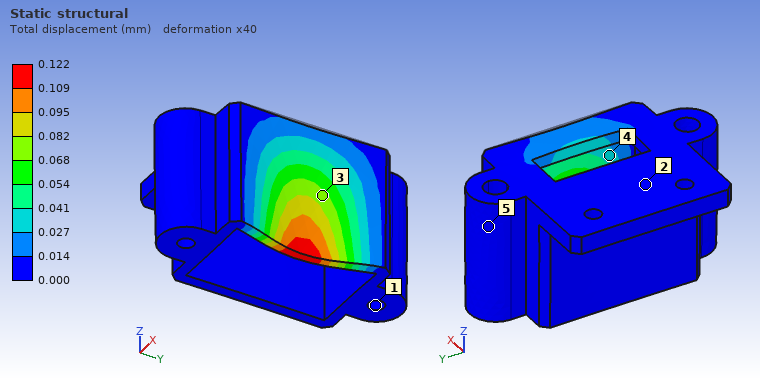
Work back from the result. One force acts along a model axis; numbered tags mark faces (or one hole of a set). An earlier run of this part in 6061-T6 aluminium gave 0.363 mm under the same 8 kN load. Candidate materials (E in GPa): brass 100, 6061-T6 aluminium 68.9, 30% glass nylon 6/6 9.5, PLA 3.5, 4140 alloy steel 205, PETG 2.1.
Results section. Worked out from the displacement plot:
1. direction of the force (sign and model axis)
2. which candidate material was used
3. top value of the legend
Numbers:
-X
4140 alloy steel
0.122 mm
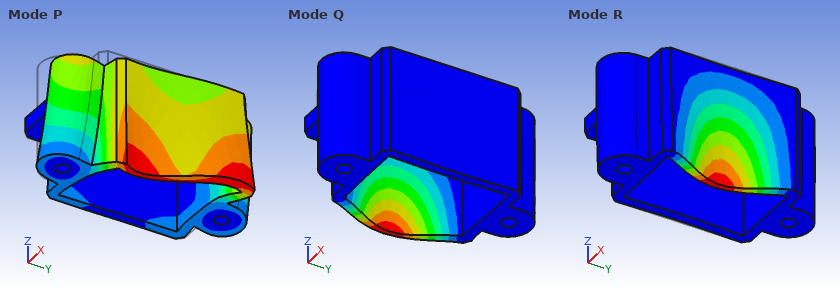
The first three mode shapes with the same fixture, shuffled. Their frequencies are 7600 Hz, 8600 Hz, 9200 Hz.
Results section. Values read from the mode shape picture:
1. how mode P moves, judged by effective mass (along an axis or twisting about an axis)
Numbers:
along Y
